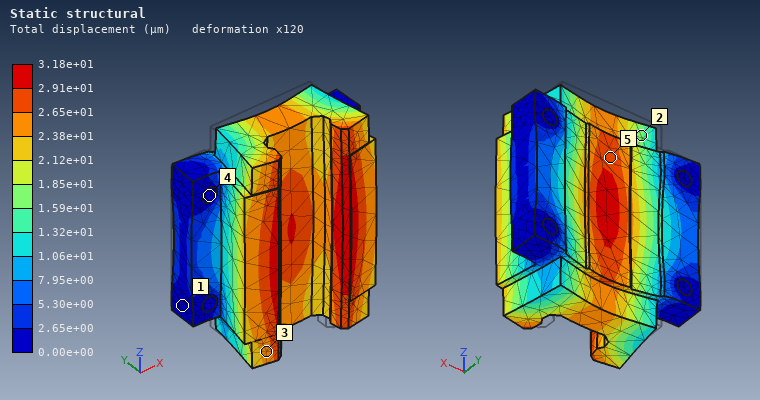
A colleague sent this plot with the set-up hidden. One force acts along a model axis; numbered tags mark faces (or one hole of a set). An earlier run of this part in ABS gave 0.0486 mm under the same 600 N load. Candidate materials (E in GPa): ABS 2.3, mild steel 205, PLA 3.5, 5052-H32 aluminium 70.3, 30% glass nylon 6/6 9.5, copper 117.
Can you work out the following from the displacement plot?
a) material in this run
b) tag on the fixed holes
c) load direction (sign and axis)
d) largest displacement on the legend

PLA
4
-Y
3.18e+01 µm
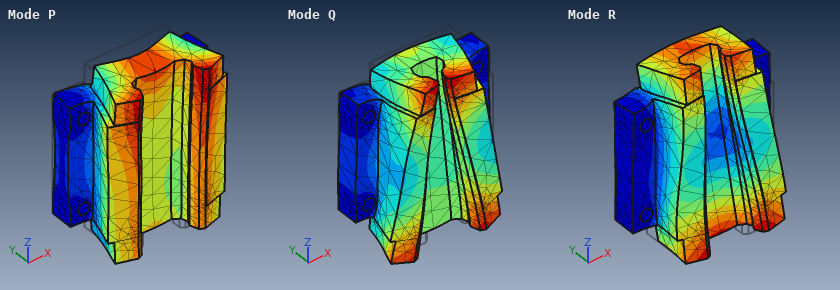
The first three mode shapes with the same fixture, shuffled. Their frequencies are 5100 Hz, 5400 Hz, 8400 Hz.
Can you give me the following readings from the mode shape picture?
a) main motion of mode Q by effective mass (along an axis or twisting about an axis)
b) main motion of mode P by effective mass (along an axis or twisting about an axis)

along Z
along Y
